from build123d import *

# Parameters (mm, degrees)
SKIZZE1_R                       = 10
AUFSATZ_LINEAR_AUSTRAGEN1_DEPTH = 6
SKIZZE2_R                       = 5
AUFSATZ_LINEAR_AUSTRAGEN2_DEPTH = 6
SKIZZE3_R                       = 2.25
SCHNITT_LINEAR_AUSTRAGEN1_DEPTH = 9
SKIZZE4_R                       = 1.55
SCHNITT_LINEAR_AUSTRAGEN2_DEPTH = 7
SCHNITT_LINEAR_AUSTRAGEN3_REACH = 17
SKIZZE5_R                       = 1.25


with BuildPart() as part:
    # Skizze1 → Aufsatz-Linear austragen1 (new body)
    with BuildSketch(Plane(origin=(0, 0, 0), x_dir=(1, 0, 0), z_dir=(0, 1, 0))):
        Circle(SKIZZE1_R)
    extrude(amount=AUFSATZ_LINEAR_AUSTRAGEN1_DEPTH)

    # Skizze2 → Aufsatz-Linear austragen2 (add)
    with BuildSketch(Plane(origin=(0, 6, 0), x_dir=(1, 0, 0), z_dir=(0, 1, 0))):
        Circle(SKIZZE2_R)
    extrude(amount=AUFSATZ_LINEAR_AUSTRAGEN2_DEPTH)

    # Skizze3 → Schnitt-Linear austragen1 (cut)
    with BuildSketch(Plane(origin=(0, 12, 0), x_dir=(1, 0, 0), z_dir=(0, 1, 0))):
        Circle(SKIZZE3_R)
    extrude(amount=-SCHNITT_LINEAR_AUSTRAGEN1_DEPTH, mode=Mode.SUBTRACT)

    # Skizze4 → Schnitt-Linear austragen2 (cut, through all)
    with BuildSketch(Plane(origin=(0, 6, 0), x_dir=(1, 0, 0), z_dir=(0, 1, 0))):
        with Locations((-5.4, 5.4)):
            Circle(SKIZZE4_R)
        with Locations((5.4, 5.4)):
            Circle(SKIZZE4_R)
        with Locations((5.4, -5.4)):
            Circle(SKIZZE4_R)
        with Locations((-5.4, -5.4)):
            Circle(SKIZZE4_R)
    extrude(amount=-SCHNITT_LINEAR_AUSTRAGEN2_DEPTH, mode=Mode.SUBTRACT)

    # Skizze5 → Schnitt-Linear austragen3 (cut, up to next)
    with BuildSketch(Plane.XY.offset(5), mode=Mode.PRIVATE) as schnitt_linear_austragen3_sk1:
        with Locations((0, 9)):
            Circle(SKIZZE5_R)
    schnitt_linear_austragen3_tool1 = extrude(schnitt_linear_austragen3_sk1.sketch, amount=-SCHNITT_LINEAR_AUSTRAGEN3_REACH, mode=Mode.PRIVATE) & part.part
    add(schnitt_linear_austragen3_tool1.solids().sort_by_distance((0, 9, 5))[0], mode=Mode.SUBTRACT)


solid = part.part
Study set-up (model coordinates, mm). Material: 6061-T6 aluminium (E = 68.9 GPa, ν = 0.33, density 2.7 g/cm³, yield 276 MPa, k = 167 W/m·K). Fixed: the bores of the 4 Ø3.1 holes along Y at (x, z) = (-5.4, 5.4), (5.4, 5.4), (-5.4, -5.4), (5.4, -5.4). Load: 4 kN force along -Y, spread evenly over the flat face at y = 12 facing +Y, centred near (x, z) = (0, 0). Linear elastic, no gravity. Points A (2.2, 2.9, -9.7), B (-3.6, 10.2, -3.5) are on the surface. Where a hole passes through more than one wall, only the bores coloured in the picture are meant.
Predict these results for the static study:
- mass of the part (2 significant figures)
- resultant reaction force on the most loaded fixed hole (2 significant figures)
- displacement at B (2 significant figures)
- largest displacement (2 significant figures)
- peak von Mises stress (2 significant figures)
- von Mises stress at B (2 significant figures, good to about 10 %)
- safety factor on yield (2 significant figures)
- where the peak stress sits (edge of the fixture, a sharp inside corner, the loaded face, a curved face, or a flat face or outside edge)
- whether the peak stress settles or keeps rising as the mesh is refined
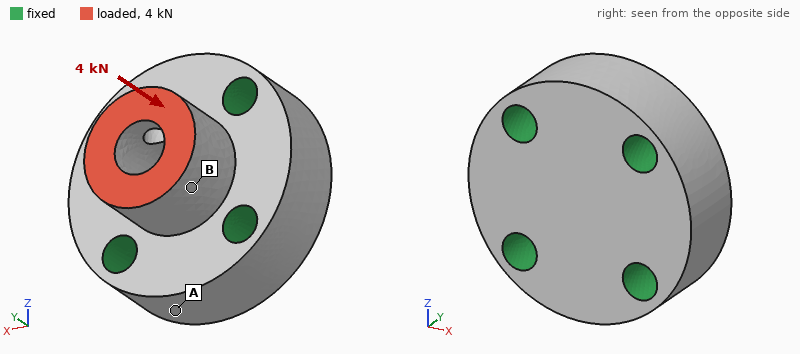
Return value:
5.4 g
1.0 kN
7.6 µm
15 µm
250 MPa
61 MPa
1.1
a curved face
settles
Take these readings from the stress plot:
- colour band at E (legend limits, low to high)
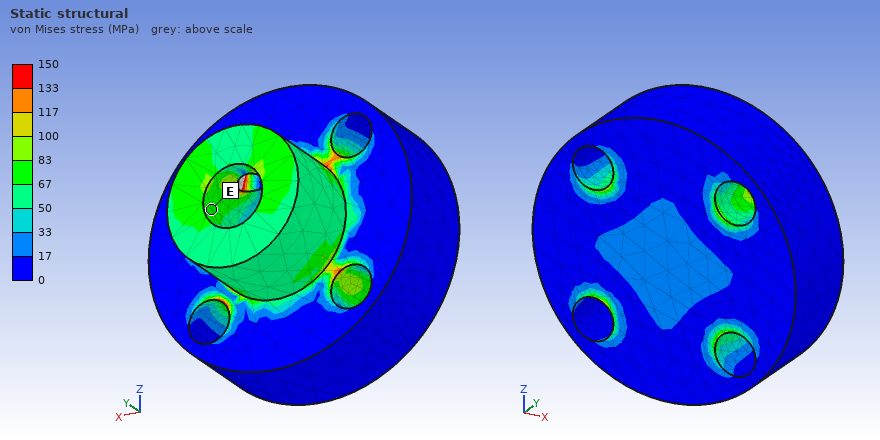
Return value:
67 to 83 MPa
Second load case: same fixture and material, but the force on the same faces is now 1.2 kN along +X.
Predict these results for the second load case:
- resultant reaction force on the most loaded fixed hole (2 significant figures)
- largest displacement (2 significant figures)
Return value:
590 N
20 µm
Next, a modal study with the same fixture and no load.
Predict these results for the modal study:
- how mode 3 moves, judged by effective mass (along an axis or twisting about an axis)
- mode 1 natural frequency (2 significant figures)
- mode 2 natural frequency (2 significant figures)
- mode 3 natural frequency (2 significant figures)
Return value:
along Y
68 kHz
71 kHz
100 kHz
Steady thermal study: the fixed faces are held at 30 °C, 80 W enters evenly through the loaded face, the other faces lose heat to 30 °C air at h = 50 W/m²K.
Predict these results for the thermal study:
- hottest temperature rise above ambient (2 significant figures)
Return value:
71 K
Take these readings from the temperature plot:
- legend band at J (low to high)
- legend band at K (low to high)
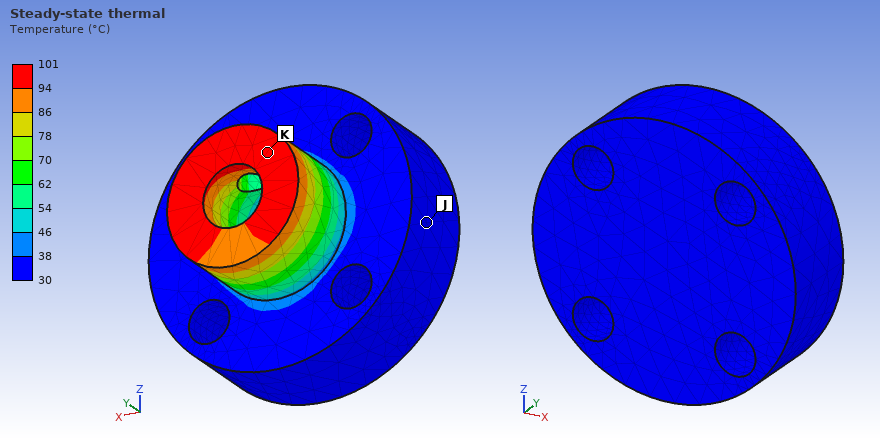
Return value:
30 to 38 °C
94 to 101 °C
